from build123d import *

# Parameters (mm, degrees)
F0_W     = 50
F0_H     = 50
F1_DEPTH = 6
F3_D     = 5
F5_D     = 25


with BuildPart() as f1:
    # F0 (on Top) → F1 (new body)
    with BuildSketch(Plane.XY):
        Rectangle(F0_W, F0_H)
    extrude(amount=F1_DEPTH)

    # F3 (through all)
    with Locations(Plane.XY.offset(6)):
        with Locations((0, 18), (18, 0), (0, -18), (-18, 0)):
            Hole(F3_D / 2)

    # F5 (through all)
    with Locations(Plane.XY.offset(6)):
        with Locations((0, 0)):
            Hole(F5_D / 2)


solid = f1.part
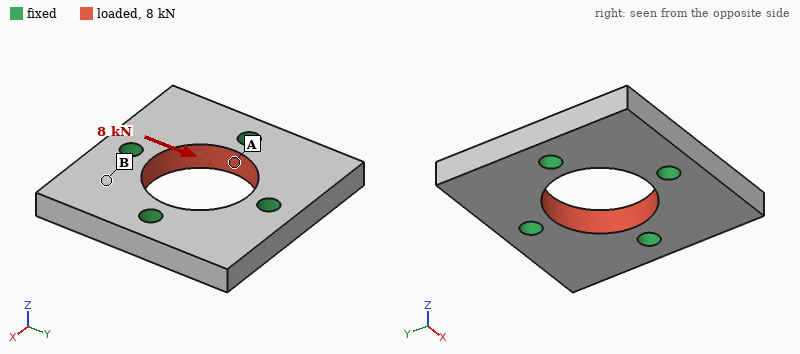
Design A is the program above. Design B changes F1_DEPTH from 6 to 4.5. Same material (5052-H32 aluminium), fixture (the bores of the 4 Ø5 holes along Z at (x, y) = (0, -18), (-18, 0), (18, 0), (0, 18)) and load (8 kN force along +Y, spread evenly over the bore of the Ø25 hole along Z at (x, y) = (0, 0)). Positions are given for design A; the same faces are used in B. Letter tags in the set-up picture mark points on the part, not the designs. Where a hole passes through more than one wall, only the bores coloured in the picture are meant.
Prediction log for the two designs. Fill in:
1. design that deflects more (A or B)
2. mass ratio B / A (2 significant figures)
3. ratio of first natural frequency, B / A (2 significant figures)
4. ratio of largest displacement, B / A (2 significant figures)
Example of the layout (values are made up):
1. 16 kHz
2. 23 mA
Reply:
1. B
2. 0.75
3. 0.80
4. 1.3
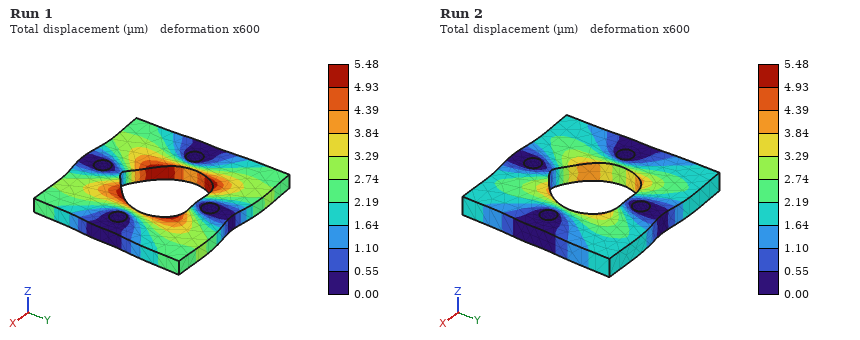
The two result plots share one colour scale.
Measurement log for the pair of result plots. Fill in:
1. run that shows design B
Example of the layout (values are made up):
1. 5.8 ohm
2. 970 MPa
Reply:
1. Run 1
